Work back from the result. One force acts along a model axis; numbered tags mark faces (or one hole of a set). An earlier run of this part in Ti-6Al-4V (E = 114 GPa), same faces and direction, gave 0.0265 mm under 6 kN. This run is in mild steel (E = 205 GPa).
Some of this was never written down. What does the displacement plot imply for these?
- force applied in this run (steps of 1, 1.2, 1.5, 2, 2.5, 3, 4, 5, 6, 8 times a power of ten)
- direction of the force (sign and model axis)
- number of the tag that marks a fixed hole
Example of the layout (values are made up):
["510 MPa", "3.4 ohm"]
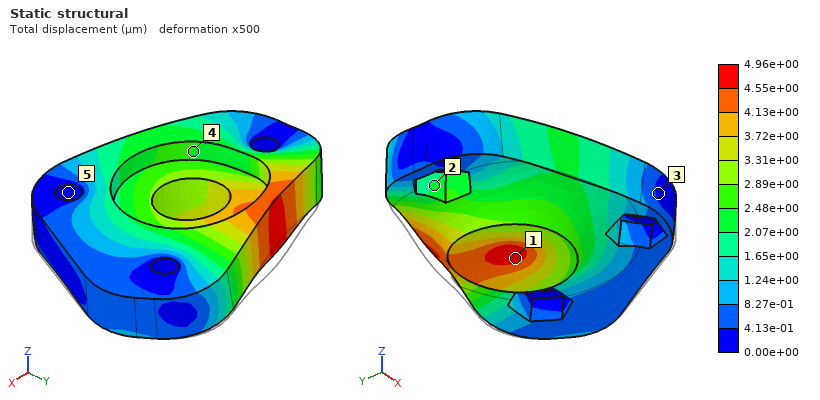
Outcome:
["2 kN", "+Z", "5"]
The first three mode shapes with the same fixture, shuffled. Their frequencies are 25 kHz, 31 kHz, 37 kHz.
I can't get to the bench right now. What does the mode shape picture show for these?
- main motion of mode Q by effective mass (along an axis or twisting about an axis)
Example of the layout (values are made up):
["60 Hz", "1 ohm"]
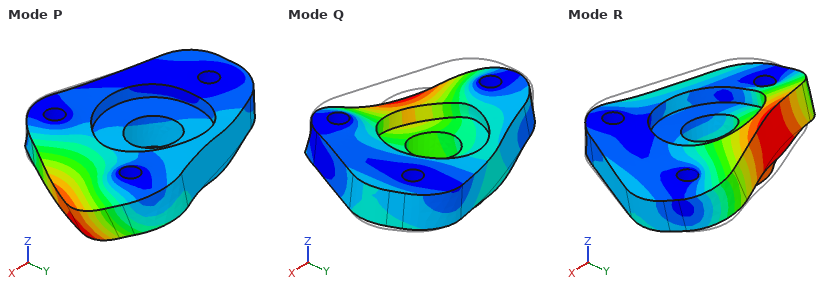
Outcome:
["along Z"]
